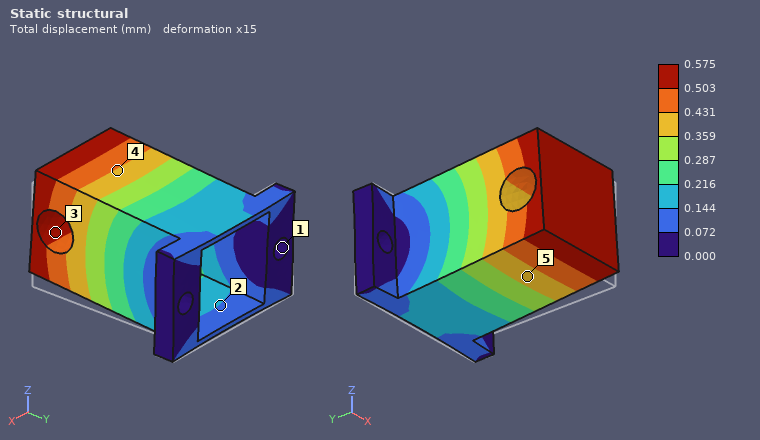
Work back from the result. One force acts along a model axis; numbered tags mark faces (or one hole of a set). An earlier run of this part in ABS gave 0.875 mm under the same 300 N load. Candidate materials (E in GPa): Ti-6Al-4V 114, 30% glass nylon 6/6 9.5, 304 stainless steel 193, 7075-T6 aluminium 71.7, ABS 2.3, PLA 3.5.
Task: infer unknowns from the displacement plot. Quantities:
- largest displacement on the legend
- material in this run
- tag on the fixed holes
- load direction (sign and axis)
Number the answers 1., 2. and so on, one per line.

1. 0.575 mm
2. PLA
3. 1
4. +Z
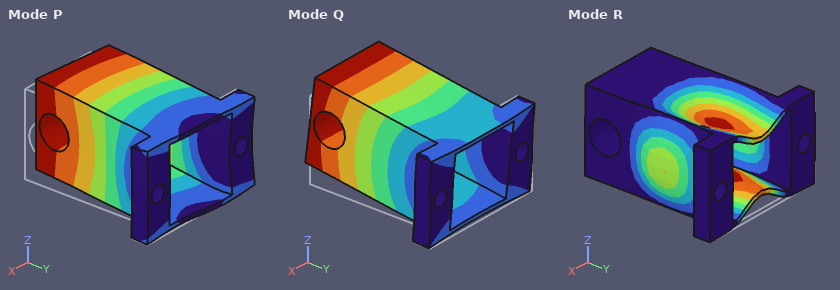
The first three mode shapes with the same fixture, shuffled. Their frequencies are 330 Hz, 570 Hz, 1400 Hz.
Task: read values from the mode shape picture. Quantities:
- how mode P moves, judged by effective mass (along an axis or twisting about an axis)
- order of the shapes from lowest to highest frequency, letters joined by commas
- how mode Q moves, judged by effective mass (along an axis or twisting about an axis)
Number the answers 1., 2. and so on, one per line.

1. along X
2. Q, P, R
3. along Z
